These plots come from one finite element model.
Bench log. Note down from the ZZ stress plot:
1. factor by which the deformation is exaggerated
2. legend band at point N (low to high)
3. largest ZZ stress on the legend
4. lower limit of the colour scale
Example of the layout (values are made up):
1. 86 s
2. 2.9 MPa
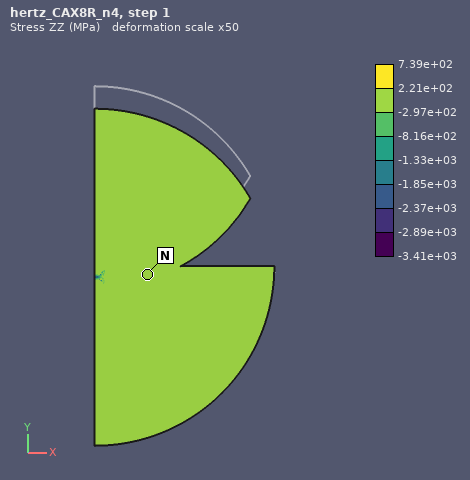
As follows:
1. 50
2. -2.97e+02 to 2.21e+02 MPa
3. 7.39e+02 MPa
4. -3.41e+03 MPa
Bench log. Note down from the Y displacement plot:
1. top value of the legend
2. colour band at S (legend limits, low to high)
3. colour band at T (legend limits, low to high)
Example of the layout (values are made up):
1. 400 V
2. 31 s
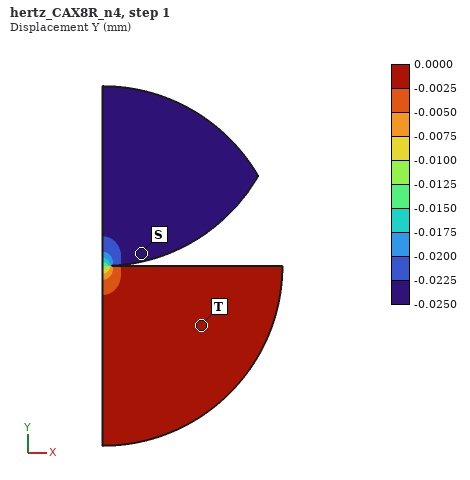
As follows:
1. 0.0000 mm
2. -0.0250 to -0.0225 mm
3. -0.0025 to 0.0000 mm
